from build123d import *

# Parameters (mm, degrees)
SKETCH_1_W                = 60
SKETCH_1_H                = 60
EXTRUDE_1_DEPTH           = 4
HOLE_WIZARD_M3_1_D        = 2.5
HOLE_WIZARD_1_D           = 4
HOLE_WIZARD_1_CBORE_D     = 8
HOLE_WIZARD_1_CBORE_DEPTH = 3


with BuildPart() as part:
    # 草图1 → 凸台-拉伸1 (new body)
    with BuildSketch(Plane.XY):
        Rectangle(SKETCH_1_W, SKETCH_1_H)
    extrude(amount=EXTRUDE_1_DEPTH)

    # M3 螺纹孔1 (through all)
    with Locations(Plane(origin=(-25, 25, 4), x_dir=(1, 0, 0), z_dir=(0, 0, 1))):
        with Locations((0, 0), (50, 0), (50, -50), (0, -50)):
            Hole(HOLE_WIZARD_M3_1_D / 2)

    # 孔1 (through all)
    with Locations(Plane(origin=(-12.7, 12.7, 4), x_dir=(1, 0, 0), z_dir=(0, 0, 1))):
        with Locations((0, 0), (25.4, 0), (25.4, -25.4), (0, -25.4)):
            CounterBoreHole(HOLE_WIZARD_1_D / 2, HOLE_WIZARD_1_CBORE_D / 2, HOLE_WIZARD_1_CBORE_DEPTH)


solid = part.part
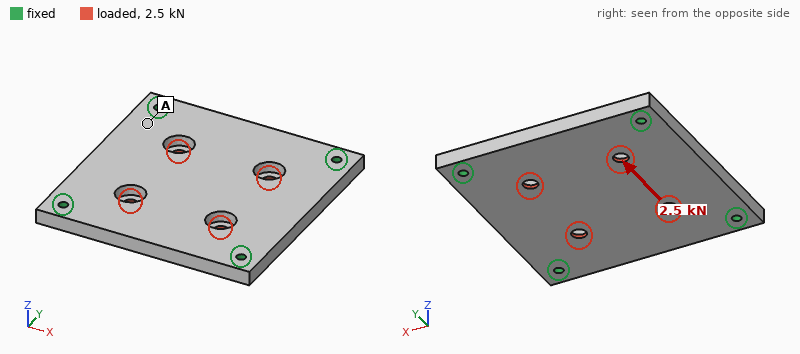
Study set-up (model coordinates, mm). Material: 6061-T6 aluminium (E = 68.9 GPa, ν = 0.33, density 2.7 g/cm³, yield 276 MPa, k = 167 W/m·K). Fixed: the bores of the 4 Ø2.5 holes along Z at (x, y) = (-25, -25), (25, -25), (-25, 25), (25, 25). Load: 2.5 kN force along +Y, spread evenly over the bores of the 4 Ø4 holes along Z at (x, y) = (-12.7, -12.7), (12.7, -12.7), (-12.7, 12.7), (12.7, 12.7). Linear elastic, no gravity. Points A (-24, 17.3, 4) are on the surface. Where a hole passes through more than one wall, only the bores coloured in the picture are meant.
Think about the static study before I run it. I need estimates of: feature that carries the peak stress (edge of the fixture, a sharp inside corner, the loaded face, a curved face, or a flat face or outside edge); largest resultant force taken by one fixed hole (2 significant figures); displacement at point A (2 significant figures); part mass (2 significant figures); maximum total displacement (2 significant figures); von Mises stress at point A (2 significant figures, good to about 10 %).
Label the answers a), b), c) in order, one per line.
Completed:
a) the loaded face
b) 670 N
c) 1.7 µm
d) 37 g
e) 8.1 µm
f) 11 MPa
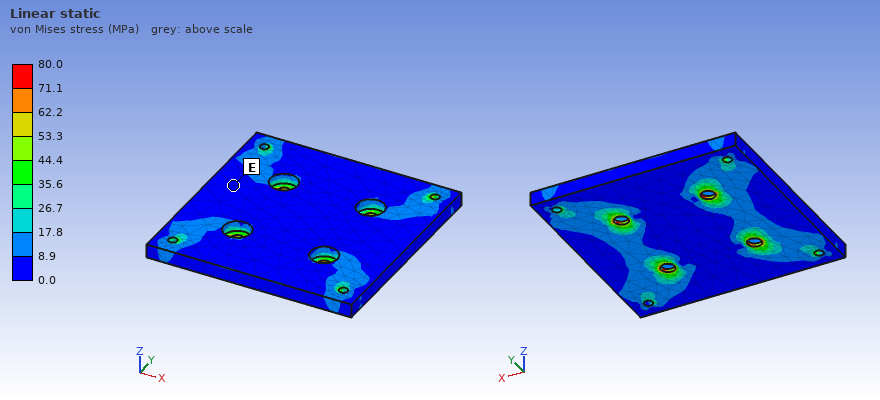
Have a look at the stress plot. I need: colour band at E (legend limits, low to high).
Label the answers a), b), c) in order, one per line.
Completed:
a) 0.0 to 8.9 MPa
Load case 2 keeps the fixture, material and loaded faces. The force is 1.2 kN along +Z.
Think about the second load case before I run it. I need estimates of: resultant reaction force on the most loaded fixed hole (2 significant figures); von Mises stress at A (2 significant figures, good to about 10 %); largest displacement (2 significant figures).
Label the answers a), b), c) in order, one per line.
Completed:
a) 310 N
b) 23 MPa
c) 67 µm
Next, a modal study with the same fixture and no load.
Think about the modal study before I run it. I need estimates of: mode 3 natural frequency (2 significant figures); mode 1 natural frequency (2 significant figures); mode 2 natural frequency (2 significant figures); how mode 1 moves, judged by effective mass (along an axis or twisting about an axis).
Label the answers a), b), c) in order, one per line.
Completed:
a) 8400 Hz
b) 5100 Hz
c) 8400 Hz
d) along Z
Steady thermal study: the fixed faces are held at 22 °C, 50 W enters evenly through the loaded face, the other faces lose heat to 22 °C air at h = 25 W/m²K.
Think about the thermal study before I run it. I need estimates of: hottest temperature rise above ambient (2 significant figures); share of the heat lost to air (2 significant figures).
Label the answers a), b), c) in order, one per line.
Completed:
a) 28 K
b) 5.2 %
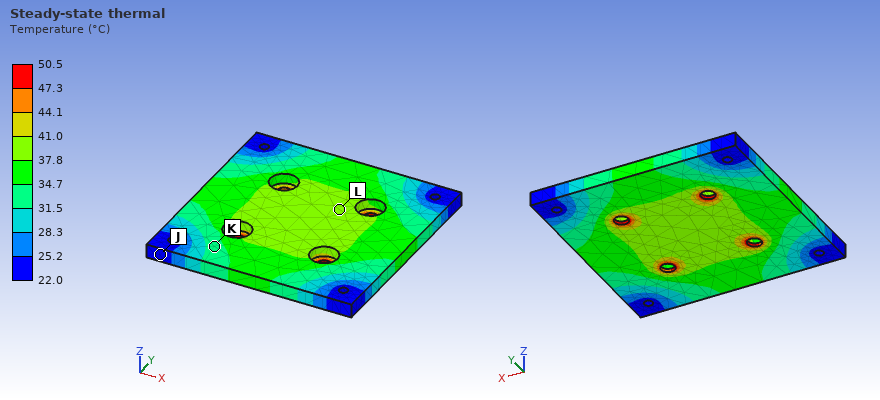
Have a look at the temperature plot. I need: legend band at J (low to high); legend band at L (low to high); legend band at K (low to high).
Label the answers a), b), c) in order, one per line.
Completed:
a) 22.0 to 25.2 °C
b) 37.8 to 41.0 °C
c) 31.5 to 34.7 °C
